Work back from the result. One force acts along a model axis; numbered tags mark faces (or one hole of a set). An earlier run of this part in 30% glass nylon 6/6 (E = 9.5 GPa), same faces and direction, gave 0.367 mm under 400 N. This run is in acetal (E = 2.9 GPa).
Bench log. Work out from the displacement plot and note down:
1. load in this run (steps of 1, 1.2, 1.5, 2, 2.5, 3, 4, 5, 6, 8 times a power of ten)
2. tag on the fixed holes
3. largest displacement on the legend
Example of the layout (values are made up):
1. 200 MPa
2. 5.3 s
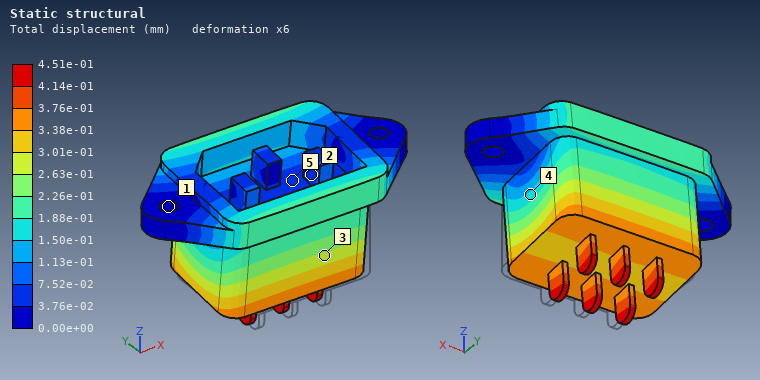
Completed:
1. 150 N
2. 1
3. 4.51e-01 mm
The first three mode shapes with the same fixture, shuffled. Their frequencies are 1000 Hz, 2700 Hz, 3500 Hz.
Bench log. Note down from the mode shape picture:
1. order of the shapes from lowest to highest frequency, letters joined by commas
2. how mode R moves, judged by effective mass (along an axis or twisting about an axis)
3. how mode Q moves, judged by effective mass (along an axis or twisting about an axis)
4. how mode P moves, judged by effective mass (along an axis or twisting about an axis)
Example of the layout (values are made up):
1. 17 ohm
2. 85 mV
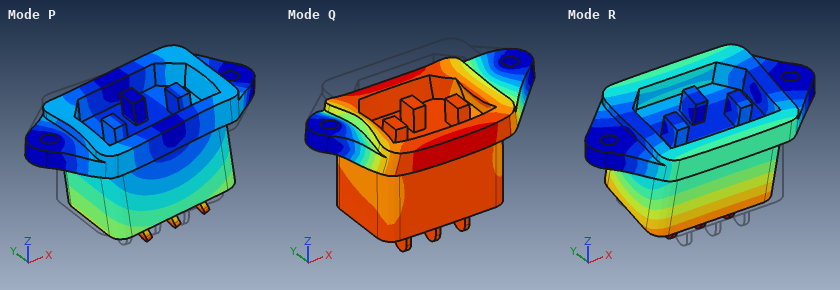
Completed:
1. R, Q, P
2. along Y
3. along Z
4. along X
